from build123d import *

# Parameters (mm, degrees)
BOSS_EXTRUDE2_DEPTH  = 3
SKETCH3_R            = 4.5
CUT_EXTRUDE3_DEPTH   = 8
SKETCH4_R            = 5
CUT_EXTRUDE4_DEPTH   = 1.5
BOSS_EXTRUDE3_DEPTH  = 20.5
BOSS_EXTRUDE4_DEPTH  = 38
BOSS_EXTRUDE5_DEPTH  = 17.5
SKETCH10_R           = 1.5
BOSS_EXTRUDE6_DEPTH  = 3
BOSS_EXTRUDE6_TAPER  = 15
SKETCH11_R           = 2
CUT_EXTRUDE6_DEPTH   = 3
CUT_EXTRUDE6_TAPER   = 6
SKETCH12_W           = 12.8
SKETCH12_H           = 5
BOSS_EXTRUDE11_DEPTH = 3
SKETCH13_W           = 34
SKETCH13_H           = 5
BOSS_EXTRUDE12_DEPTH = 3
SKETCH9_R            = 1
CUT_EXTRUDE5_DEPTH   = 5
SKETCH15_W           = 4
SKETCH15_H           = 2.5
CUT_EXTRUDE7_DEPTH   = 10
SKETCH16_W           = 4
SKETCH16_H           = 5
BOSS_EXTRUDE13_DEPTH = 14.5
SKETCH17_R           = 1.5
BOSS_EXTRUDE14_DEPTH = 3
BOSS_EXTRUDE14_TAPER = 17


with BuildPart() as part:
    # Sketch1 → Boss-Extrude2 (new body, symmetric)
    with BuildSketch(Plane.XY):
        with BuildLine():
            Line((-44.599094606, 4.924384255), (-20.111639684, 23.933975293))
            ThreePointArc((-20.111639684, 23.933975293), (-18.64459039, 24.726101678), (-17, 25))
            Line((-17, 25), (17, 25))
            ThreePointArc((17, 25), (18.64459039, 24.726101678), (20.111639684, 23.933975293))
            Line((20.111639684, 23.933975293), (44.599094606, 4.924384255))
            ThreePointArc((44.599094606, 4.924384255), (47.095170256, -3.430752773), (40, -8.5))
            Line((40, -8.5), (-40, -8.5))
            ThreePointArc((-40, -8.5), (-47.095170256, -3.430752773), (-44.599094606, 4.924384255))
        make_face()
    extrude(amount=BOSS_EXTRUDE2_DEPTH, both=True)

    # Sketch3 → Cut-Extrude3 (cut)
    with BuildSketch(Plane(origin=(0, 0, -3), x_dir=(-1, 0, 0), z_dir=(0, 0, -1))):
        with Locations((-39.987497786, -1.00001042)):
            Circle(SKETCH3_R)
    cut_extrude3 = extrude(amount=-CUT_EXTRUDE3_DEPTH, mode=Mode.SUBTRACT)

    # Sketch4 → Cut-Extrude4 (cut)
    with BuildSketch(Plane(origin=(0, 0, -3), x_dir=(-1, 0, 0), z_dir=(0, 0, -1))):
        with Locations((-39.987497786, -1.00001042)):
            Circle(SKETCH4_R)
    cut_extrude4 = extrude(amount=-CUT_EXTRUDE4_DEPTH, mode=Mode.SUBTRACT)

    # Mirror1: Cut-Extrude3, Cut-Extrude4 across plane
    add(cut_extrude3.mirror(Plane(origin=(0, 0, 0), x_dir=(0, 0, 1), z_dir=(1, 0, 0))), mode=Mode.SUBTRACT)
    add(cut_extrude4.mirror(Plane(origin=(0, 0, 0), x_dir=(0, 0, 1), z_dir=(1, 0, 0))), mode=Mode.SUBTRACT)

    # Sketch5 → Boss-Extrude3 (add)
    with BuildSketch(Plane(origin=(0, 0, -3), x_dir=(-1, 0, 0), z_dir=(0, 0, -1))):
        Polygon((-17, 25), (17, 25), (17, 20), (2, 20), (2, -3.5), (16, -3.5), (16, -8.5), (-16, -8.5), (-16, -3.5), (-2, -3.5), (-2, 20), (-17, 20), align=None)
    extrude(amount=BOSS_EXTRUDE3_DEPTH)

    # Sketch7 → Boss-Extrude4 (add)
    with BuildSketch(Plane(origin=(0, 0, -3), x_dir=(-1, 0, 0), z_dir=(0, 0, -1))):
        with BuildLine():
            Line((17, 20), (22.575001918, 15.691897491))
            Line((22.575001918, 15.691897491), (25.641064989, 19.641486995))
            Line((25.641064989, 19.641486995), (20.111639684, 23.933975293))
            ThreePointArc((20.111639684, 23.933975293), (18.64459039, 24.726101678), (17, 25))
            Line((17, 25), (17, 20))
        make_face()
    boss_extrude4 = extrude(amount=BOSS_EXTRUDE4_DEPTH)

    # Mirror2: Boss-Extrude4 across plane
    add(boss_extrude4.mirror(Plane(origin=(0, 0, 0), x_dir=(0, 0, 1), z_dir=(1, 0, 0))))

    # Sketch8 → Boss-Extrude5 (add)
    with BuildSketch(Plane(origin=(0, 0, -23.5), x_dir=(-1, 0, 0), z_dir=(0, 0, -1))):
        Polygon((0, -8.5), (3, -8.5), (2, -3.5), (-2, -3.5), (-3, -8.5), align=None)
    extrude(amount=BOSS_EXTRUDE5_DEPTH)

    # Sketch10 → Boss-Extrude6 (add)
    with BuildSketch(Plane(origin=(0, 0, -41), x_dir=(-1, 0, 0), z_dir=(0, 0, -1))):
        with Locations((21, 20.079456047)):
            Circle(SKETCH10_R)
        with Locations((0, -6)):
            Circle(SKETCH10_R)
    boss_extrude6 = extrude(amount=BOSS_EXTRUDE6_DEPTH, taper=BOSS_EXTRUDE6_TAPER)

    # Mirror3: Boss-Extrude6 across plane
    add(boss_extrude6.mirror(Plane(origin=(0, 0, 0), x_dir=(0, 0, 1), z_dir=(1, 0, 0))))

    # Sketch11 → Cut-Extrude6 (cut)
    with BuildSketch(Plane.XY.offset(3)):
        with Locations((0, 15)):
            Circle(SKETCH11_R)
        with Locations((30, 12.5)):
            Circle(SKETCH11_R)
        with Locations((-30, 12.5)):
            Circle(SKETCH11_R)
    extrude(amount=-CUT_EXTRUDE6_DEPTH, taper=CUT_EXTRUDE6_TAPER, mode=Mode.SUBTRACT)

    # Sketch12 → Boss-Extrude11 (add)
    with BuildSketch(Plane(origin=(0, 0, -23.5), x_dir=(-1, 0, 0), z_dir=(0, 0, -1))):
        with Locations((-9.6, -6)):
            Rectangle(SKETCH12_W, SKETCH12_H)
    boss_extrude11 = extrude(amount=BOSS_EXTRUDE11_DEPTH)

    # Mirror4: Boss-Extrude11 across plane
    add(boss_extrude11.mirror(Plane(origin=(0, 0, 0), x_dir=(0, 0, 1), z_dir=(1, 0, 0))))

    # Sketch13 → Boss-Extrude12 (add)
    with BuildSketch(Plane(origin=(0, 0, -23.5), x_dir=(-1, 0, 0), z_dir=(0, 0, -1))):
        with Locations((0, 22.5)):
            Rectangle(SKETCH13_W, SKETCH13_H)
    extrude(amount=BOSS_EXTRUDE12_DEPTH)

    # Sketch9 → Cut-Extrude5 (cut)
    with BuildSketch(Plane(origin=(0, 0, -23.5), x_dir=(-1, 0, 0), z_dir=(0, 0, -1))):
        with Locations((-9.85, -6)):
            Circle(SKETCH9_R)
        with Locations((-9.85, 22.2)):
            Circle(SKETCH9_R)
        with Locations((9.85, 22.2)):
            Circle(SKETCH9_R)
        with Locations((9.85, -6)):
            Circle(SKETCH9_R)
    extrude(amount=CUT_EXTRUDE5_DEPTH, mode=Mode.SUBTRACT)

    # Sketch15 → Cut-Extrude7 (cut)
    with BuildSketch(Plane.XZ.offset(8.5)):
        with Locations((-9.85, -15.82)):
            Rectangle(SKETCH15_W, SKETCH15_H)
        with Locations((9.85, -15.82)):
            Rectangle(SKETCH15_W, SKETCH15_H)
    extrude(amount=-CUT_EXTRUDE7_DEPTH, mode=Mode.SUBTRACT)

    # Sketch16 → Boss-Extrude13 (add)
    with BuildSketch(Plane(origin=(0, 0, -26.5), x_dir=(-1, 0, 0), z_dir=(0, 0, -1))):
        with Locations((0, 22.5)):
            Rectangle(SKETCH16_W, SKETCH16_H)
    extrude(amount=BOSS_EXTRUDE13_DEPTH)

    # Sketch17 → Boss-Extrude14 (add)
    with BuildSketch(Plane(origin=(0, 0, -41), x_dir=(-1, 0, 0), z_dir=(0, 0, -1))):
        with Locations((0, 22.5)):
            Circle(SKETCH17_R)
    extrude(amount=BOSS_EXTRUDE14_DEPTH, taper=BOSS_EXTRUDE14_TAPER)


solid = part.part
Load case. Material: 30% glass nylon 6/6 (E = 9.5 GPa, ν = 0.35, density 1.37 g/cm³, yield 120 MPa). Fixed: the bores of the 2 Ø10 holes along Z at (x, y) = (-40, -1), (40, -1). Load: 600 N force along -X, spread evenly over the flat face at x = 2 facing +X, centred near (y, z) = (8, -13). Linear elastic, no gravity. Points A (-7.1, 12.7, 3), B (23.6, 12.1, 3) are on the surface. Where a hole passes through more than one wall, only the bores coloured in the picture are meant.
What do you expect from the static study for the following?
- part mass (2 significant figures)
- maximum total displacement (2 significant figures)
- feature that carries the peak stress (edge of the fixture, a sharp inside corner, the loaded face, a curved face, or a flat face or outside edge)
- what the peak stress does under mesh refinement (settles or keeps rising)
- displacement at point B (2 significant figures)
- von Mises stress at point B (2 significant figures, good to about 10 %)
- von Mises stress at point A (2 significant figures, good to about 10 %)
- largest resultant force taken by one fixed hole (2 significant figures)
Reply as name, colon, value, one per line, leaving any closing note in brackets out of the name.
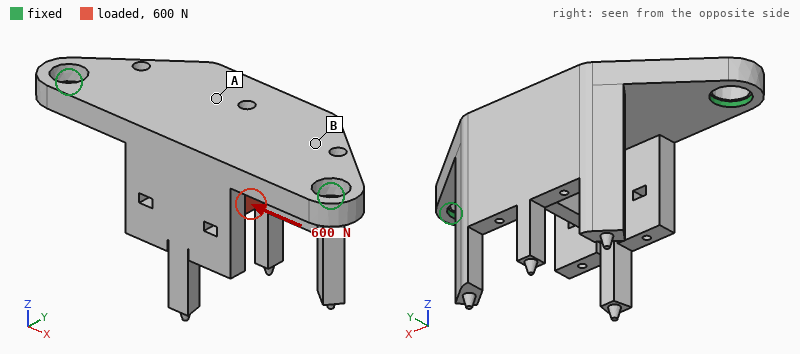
part mass: 38 g
maximum total displacement: 0.18 mm
feature that carries the peak stress: edge of the fixture
what the peak stress does under mesh refinement: keeps rising
displacement at point B: 0.043 mm
von Mises stress at point B: 6.8 MPa
von Mises stress at point A: 2.0 MPa
largest resultant force taken by one fixed hole: 330 N
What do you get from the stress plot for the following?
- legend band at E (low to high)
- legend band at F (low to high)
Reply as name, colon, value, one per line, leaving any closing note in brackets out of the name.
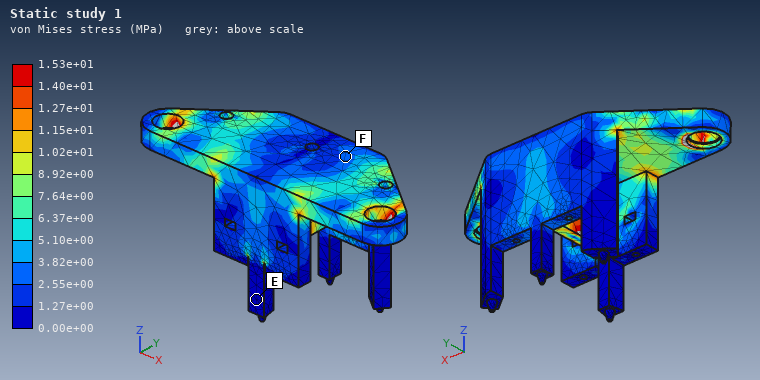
legend band at E: 0.00e+00 to 1.27e+00 MPa
legend band at F: 2.55e+00 to 3.82e+00 MPa
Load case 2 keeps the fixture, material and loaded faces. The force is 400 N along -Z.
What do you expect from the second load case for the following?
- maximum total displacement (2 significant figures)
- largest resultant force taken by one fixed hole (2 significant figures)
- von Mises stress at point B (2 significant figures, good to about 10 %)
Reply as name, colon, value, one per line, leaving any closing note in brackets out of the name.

maximum total displacement: 0.35 mm
largest resultant force taken by one fixed hole: 250 N
von Mises stress at point B: 11 MPa
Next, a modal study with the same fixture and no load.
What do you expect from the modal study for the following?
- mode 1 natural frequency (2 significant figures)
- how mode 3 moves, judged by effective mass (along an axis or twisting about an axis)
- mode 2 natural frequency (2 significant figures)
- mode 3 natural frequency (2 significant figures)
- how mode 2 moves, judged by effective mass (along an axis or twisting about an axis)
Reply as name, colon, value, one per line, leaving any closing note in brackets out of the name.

mode 1 natural frequency: 860 Hz
how mode 3 moves, judged by effective mass: along X
mode 2 natural frequency: 1900 Hz
mode 3 natural frequency: 2000 Hz
how mode 2 moves, judged by effective mass: along Z
